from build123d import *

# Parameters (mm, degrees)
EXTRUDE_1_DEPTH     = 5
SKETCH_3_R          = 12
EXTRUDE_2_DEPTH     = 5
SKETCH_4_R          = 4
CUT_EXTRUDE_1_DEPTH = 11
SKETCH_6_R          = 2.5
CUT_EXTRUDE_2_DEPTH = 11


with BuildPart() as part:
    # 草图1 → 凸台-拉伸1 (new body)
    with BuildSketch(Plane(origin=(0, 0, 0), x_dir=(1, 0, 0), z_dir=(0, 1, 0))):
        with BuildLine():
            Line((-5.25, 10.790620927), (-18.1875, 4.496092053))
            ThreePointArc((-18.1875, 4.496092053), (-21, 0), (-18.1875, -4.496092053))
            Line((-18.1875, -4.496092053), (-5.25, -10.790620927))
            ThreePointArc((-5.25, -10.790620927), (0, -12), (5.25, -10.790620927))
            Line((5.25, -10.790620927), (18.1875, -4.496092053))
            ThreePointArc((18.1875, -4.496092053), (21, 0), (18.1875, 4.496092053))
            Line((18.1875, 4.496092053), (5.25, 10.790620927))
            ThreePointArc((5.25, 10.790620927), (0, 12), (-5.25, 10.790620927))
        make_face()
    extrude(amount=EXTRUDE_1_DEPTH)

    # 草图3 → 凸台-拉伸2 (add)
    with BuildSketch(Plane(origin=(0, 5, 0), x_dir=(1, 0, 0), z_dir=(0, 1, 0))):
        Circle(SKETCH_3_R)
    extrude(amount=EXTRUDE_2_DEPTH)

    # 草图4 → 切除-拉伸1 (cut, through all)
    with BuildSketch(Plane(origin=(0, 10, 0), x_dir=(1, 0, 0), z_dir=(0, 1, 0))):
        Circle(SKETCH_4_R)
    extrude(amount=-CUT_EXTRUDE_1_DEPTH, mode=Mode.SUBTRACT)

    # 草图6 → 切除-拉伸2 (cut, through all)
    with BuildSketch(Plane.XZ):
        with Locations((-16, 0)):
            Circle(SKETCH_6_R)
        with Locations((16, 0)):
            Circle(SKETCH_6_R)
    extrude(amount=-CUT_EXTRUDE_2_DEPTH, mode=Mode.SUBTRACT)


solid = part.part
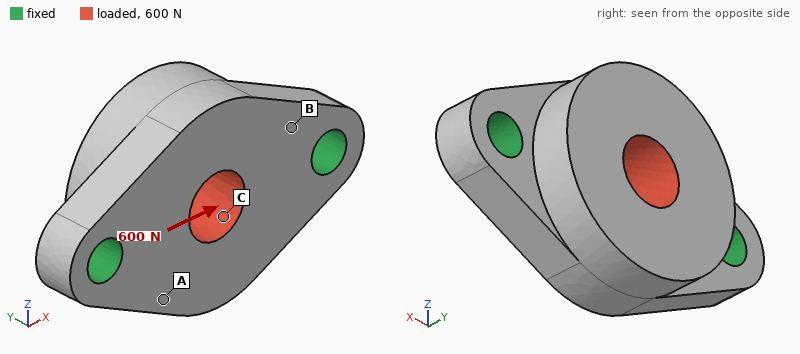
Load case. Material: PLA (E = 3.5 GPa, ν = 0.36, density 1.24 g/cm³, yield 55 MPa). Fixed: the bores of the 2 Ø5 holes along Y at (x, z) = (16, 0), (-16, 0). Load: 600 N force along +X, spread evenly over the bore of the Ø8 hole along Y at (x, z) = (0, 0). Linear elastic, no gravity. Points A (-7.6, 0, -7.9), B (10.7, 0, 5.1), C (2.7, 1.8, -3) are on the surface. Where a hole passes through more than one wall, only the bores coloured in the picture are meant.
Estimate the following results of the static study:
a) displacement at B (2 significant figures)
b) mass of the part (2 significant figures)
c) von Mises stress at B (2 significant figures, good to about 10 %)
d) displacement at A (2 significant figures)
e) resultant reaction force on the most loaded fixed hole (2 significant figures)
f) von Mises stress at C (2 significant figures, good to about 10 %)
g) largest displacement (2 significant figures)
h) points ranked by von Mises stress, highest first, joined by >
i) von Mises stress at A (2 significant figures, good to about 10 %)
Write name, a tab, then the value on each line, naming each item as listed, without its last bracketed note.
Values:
displacement at B	8.0 µm
mass of the part	6.1 g
von Mises stress at B	2.0 MPa
displacement at A	9.8 µm
resultant reaction force on the most loaded fixed hole	300 N
von Mises stress at C	3.8 MPa
largest displacement	18 µm
points ranked by von Mises stress, highest first, joined by >	C > B > A
von Mises stress at A	1.2 MPa
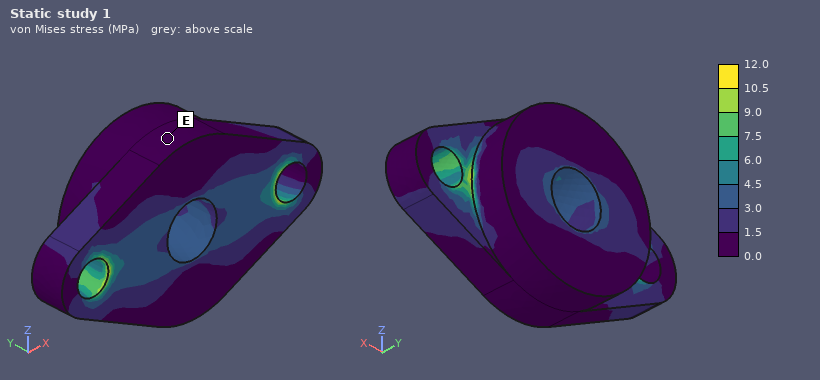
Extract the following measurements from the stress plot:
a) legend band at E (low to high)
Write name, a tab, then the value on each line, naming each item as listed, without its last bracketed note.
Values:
legend band at E	0.0 to 1.5 MPa
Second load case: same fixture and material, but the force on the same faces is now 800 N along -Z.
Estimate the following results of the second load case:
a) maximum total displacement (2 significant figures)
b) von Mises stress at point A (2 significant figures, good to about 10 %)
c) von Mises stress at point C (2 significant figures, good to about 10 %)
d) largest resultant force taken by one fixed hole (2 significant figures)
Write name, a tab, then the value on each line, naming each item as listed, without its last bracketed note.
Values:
maximum total displacement	0.13 mm
von Mises stress at point A	7.6 MPa
von Mises stress at point C	4.7 MPa
largest resultant force taken by one fixed hole	400 N
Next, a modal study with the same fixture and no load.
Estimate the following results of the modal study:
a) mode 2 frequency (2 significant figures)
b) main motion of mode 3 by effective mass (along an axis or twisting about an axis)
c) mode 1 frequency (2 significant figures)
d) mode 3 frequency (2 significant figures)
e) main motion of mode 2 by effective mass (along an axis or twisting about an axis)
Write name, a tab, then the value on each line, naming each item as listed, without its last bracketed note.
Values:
mode 2 frequency	7400 Hz
main motion of mode 3 by effective mass	along Z
mode 1 frequency	4900 Hz
mode 3 frequency	11 kHz
main motion of mode 2 by effective mass	along Y
